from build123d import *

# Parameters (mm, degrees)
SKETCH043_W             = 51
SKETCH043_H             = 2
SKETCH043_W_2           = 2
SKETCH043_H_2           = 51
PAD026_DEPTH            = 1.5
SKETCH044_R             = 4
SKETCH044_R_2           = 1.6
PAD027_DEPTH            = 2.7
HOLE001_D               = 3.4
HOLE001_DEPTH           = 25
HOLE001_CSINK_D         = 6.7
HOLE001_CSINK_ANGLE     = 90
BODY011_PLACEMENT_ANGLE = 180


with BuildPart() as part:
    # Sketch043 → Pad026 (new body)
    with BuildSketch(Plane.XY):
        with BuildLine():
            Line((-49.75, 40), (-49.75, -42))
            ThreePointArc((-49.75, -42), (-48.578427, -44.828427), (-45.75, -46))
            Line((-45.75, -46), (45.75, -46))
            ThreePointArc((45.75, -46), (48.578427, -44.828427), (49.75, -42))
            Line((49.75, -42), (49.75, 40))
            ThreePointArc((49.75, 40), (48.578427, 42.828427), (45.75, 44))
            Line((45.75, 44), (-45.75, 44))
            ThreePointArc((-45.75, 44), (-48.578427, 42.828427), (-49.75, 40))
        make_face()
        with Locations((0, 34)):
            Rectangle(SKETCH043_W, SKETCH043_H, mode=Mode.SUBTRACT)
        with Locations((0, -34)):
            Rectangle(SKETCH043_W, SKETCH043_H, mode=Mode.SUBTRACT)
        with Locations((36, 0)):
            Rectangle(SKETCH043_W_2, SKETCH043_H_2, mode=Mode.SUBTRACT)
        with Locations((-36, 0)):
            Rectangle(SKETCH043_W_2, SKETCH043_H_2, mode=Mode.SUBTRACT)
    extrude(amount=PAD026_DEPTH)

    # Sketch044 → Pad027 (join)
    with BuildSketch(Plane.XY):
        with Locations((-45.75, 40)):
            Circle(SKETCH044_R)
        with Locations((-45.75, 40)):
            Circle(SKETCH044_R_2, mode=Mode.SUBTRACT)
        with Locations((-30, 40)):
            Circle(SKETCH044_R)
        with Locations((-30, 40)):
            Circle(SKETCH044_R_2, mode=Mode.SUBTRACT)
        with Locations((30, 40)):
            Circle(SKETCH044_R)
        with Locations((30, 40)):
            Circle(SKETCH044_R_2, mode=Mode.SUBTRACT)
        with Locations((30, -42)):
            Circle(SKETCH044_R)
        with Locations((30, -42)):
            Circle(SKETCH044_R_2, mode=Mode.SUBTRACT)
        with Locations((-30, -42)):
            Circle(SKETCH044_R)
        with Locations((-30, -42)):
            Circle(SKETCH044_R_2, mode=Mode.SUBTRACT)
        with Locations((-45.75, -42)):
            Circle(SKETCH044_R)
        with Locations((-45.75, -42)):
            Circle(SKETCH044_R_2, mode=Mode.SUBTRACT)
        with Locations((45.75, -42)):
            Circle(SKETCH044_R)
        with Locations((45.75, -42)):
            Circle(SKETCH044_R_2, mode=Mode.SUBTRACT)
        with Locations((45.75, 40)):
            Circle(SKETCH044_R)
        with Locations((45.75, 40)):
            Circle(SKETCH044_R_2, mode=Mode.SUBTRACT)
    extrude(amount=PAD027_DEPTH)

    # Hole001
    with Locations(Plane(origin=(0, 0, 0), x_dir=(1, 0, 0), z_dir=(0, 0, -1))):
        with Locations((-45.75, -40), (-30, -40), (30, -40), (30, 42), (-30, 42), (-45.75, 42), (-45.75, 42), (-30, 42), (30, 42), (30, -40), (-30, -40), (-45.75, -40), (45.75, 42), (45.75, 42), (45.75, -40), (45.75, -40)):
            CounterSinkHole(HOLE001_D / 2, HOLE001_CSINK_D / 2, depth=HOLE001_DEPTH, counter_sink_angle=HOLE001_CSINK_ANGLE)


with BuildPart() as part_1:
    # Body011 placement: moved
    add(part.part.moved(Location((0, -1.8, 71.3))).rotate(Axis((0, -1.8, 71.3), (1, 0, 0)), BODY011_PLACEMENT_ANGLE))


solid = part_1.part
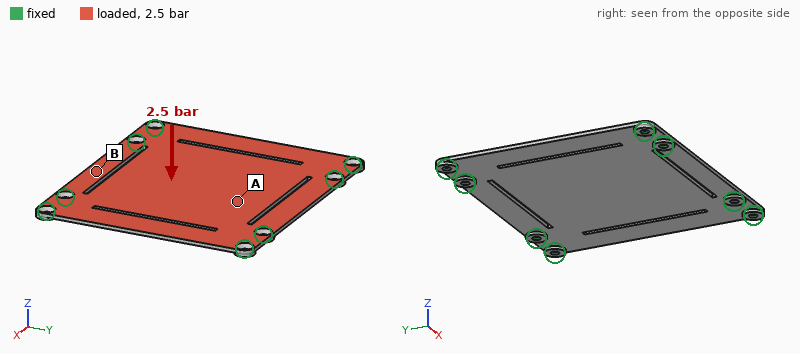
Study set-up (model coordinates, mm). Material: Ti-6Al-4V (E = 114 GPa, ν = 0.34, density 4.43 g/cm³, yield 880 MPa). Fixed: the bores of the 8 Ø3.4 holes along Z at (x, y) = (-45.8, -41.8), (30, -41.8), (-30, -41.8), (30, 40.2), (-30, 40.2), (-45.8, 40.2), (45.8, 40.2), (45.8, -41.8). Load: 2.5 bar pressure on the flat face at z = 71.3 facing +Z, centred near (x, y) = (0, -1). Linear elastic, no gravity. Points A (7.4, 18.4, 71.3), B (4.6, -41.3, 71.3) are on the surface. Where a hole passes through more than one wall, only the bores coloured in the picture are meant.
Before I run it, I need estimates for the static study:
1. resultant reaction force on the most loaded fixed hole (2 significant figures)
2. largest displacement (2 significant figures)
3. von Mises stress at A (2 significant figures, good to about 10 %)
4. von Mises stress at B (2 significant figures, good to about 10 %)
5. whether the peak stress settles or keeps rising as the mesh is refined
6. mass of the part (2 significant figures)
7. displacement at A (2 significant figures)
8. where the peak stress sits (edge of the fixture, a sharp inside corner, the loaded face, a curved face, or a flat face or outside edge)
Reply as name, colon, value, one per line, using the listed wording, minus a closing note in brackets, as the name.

resultant reaction force on the most loaded fixed hole: 900 N
largest displacement: 1.5 mm
von Mises stress at A: 150 MPa
von Mises stress at B: 76 MPa
whether the peak stress settles or keeps rising as the mesh is refined: keeps rising
mass of the part: 57 g
displacement at A: 1.1 mm
where the peak stress sits: edge of the fixture
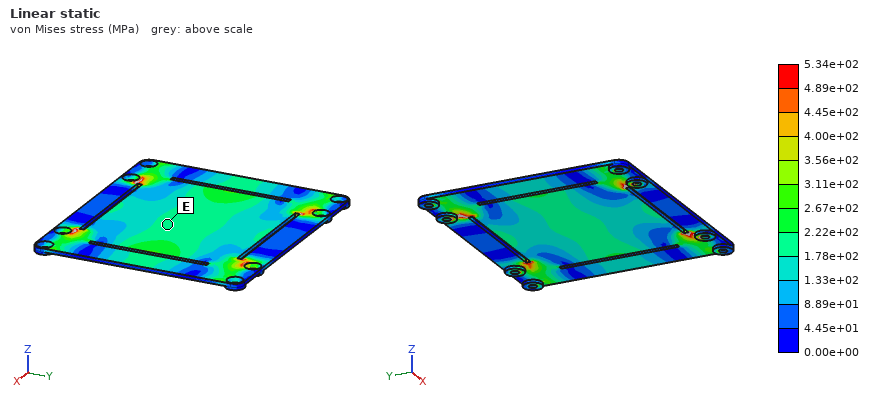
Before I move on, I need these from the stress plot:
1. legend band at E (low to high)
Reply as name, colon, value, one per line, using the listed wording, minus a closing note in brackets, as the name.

legend band at E: 1.78e+02 to 2.22e+02 MPa
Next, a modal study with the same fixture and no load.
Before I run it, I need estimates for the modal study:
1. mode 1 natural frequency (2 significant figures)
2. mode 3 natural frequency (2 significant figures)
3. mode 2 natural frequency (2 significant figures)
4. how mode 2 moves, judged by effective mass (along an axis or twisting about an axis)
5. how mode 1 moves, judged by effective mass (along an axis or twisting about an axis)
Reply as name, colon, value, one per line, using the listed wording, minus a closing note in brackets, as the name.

mode 1 natural frequency: 950 Hz
mode 3 natural frequency: 1500 Hz
mode 2 natural frequency: 1400 Hz
how mode 2 moves, judged by effective mass: twisting about Y
how mode 1 moves, judged by effective mass: along Z
